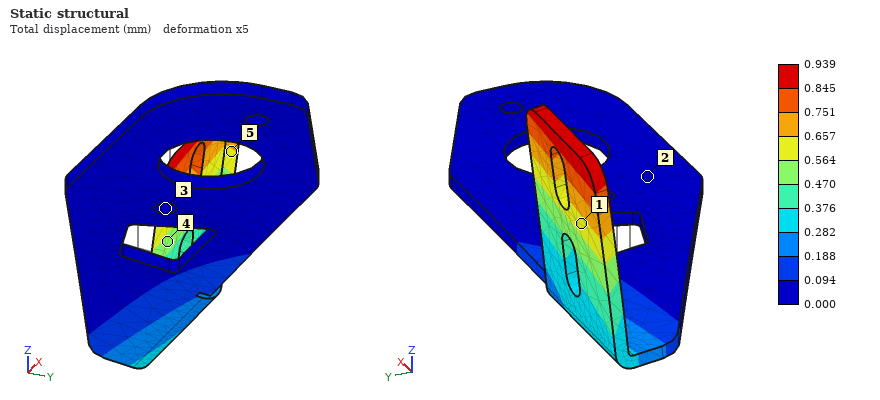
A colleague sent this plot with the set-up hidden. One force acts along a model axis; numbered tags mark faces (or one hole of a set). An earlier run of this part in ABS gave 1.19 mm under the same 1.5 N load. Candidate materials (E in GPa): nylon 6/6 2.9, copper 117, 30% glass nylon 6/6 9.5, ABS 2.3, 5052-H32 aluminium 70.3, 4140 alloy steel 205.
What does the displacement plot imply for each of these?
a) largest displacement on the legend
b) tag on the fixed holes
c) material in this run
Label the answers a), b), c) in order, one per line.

a) 0.939 mm
b) 3
c) nylon 6/6
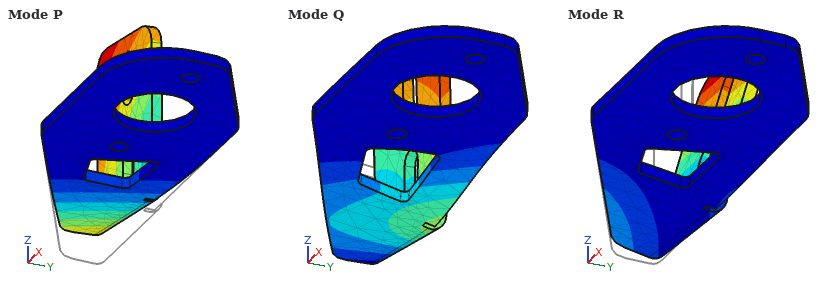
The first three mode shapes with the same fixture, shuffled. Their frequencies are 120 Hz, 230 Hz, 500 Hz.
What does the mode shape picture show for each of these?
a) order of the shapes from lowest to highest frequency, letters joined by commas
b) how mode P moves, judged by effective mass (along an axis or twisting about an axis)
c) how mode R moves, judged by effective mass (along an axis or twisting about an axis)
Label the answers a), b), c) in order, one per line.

a) P, R, Q
b) along Z
c) along Y
